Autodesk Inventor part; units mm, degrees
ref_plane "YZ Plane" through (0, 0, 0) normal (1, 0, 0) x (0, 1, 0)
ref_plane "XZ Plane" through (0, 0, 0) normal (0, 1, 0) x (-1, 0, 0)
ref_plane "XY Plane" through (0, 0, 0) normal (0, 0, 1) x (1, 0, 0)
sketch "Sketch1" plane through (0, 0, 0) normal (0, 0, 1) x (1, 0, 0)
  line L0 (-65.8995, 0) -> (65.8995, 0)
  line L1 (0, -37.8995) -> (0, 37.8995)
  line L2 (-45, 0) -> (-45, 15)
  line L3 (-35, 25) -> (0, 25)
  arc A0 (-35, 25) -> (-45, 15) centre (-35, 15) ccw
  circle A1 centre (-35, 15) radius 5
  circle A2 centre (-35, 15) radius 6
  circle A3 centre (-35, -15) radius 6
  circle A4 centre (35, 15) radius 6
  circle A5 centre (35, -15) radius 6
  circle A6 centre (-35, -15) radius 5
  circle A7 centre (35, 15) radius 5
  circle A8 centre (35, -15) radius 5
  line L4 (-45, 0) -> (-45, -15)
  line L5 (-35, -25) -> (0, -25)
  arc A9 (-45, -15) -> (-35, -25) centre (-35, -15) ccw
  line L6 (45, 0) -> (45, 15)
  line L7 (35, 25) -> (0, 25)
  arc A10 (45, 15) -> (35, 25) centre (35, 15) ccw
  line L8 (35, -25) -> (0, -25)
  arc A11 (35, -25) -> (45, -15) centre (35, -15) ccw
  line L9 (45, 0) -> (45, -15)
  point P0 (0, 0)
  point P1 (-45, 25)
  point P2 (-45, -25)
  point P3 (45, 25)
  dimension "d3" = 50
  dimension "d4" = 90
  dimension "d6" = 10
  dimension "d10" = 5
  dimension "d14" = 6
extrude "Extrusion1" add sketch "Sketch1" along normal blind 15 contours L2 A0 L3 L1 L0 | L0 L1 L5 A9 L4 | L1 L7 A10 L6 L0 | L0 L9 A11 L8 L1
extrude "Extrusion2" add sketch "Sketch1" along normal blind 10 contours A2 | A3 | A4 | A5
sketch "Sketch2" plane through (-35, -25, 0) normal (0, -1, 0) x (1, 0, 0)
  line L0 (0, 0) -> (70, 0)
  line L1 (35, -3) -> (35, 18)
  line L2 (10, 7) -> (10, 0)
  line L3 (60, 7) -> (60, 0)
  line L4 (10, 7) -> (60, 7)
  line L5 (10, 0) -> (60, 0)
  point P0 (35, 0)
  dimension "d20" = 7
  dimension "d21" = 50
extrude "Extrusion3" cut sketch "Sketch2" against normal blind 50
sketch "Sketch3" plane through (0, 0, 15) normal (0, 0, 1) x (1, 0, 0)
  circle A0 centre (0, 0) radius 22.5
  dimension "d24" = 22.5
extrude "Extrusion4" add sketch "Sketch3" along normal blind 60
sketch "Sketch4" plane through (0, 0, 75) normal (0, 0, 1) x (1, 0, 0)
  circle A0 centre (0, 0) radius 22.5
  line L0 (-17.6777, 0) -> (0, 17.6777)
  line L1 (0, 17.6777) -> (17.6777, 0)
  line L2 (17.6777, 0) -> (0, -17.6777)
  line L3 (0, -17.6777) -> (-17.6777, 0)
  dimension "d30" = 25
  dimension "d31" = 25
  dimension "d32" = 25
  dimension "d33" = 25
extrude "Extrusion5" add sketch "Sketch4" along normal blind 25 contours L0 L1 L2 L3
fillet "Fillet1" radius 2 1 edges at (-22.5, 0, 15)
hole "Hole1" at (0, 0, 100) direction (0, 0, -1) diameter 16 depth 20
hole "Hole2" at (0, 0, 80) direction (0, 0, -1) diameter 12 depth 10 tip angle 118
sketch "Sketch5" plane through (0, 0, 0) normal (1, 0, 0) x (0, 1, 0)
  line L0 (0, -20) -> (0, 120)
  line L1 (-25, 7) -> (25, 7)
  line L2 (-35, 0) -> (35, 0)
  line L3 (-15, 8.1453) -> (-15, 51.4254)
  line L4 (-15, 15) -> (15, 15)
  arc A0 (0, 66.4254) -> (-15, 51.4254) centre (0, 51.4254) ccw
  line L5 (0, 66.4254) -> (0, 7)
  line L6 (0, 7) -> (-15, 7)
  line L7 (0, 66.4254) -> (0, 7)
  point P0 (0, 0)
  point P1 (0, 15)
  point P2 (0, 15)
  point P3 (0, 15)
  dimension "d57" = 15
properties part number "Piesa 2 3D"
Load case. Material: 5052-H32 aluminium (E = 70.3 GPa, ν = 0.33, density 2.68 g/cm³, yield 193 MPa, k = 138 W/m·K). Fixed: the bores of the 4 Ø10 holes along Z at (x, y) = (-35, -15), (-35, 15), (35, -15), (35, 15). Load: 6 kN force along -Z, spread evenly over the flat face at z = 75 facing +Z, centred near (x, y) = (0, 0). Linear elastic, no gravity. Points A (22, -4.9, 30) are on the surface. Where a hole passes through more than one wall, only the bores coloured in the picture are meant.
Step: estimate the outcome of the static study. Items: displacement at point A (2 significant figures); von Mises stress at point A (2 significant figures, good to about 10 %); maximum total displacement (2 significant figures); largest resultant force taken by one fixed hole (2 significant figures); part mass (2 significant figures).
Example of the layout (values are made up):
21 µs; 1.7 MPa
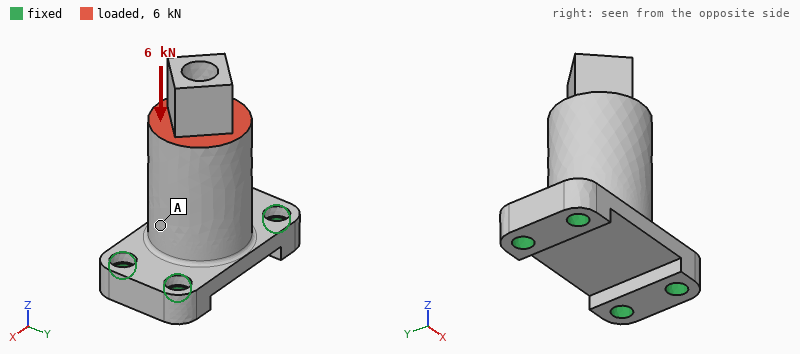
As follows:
9.8 µm; 5.6 MPa; 13 µm; 2.0 kN; 400 g
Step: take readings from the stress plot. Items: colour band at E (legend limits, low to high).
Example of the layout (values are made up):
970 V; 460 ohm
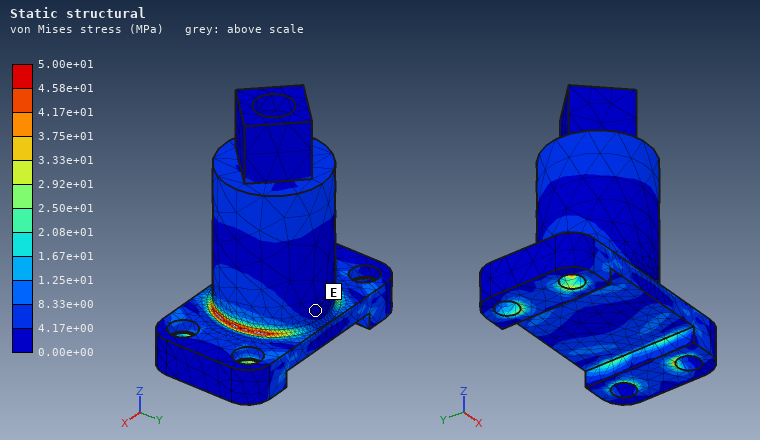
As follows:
0.00e+00 to 4.17e+00 MPa
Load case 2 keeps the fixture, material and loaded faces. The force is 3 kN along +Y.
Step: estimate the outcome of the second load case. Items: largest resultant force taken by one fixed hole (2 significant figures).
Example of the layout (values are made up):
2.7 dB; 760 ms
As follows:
4.0 kN
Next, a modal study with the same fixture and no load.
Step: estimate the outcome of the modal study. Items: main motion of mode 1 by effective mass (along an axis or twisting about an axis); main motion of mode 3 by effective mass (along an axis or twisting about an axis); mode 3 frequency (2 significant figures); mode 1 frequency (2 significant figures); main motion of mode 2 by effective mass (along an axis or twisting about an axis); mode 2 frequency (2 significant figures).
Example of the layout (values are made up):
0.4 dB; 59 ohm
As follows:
along Y; along Z; 6700 Hz; 2100 Hz; along X; 3500 Hz
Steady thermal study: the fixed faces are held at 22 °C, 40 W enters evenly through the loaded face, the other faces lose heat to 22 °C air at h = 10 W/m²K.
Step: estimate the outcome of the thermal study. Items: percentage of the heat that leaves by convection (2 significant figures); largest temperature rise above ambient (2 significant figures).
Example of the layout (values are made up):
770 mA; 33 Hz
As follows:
5.0 %; 18 K
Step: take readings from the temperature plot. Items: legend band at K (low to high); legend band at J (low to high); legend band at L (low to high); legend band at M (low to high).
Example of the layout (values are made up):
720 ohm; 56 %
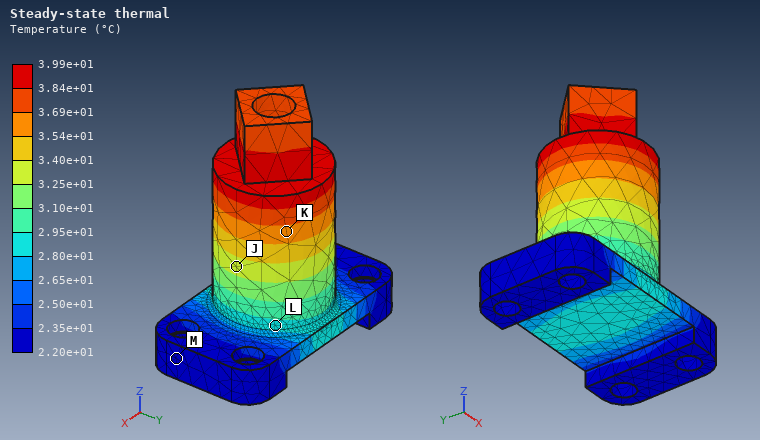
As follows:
3.54e+01 to 3.69e+01 °C; 3.25e+01 to 3.40e+01 °C; 2.80e+01 to 2.95e+01 °C; 2.20e+01 to 2.35e+01 °C
